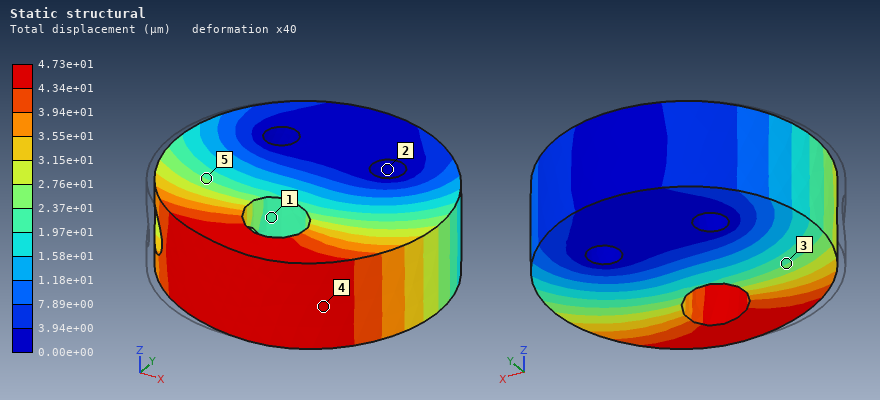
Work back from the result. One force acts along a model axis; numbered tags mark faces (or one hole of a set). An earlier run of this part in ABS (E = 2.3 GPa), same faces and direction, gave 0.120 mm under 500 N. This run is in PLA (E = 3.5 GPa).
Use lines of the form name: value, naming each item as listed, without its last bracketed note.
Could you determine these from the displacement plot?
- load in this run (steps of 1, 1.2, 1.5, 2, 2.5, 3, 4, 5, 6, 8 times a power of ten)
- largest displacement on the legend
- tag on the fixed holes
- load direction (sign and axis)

load in this run: 300 N
largest displacement on the legend: 4.73e+01 µm
tag on the fixed holes: 2
load direction: +X
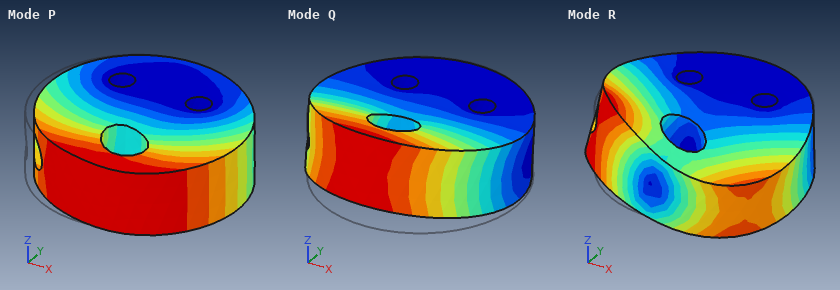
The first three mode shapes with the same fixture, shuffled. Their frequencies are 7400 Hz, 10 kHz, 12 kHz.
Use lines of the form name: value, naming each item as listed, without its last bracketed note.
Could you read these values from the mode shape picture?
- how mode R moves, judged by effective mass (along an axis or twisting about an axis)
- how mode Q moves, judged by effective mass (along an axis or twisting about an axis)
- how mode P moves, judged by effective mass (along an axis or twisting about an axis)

how mode R moves, judged by effective mass: twisting about Y
how mode Q moves, judged by effective mass: along Z
how mode P moves, judged by effective mass: along X
